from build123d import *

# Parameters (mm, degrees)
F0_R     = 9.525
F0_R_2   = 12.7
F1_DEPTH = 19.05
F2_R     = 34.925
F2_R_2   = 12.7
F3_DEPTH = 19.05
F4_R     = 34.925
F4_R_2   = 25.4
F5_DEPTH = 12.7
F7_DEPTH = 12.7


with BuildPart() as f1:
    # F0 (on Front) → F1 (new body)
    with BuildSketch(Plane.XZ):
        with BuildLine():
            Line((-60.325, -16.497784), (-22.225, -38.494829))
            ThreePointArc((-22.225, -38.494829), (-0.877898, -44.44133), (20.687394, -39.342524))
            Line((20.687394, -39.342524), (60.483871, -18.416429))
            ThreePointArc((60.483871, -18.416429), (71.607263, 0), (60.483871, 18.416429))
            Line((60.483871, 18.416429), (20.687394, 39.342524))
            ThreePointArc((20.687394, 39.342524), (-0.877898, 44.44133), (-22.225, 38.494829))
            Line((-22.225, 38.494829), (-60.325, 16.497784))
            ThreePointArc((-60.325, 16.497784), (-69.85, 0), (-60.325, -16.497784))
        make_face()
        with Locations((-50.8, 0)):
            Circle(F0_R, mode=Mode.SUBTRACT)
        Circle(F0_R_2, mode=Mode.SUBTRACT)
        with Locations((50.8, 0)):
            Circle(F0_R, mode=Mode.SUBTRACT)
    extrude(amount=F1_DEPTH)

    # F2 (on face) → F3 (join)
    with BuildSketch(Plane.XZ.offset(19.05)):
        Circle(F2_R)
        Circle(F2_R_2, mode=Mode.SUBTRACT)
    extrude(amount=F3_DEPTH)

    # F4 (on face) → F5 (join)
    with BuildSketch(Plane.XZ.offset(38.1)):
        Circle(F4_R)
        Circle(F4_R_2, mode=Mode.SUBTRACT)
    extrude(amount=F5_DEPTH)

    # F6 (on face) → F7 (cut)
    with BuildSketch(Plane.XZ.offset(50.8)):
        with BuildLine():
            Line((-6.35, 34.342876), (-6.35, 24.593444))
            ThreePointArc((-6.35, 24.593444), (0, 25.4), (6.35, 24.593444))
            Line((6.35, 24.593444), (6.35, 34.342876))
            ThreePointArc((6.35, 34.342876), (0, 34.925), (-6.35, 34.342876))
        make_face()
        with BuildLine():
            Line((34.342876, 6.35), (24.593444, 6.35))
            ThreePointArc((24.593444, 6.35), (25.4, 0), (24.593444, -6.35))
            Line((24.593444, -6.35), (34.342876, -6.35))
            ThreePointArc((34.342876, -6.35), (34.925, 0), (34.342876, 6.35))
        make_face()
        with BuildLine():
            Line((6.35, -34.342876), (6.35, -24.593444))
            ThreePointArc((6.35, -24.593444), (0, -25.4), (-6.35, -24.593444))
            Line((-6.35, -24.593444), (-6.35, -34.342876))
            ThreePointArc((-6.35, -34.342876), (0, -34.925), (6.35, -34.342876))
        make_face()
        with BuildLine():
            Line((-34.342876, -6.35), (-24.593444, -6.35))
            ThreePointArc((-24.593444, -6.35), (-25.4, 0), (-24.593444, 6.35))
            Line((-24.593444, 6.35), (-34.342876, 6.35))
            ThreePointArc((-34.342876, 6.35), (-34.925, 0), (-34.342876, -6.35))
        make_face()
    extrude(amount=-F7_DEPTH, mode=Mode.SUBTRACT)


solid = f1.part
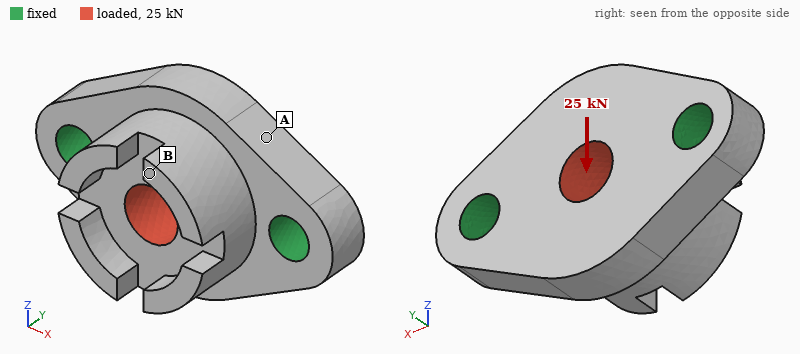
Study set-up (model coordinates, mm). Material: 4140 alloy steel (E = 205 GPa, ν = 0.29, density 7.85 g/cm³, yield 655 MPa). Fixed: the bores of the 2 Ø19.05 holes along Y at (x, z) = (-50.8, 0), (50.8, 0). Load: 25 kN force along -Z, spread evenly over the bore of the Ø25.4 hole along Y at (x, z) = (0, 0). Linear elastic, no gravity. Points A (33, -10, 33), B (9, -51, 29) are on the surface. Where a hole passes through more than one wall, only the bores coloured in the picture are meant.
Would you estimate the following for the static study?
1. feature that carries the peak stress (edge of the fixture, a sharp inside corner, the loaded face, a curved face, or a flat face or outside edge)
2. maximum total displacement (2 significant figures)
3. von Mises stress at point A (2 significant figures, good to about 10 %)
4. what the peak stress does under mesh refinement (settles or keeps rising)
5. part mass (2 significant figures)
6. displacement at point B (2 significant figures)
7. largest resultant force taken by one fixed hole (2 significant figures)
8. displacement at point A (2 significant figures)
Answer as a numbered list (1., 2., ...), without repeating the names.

1. edge of the fixture
2. 17 µm
3. 20 MPa
4. keeps rising
5. 1.7 kg
6. 17 µm
7. 13 kN
8. 7.0 µm
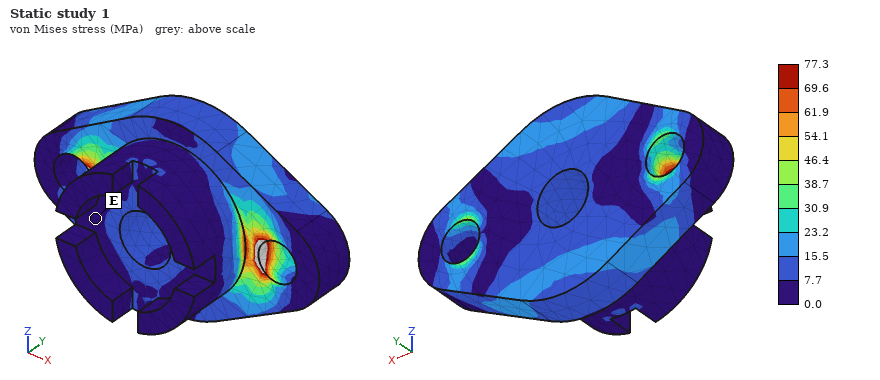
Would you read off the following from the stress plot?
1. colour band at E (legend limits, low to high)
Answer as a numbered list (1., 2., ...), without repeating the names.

1. 0.0 to 7.7 MPa
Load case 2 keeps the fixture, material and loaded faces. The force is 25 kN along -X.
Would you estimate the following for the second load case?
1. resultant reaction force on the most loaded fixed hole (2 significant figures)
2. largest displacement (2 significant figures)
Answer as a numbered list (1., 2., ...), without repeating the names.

1. 13 kN
2. 3.8 µm
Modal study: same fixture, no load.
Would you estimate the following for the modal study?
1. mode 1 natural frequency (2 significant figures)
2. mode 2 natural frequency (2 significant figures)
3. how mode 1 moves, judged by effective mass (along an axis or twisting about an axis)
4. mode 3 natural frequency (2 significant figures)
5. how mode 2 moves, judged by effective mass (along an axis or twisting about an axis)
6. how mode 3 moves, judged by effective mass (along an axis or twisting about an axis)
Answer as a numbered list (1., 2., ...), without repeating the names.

1. 4700 Hz
2. 7300 Hz
3. along Z
4. 11 kHz
5. along Y
6. along Z
